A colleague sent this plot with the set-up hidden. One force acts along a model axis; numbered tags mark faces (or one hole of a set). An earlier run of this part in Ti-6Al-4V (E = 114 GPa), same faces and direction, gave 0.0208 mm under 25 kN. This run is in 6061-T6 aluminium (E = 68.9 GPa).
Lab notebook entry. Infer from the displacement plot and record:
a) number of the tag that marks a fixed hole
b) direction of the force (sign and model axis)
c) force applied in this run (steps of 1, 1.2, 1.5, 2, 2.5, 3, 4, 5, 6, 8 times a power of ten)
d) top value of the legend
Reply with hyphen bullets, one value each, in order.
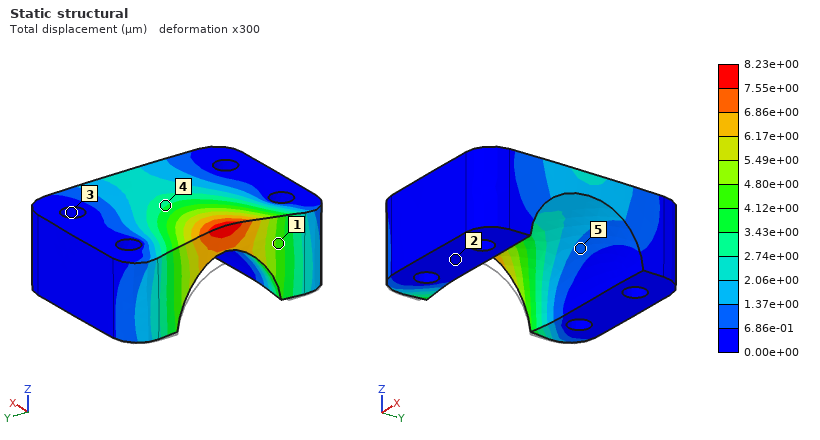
- 3
- +X
- 6 kN
- 8.23e+00 µm
